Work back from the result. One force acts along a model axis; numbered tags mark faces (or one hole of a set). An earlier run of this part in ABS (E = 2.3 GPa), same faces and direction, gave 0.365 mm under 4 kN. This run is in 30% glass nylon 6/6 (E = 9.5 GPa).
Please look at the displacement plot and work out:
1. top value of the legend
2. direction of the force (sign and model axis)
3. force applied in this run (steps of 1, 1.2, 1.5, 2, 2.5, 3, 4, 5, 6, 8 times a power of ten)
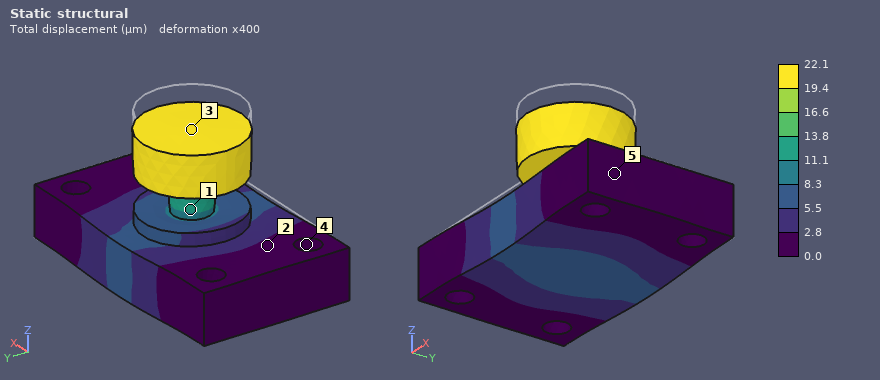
22.1 µm
-Z
1 kN
